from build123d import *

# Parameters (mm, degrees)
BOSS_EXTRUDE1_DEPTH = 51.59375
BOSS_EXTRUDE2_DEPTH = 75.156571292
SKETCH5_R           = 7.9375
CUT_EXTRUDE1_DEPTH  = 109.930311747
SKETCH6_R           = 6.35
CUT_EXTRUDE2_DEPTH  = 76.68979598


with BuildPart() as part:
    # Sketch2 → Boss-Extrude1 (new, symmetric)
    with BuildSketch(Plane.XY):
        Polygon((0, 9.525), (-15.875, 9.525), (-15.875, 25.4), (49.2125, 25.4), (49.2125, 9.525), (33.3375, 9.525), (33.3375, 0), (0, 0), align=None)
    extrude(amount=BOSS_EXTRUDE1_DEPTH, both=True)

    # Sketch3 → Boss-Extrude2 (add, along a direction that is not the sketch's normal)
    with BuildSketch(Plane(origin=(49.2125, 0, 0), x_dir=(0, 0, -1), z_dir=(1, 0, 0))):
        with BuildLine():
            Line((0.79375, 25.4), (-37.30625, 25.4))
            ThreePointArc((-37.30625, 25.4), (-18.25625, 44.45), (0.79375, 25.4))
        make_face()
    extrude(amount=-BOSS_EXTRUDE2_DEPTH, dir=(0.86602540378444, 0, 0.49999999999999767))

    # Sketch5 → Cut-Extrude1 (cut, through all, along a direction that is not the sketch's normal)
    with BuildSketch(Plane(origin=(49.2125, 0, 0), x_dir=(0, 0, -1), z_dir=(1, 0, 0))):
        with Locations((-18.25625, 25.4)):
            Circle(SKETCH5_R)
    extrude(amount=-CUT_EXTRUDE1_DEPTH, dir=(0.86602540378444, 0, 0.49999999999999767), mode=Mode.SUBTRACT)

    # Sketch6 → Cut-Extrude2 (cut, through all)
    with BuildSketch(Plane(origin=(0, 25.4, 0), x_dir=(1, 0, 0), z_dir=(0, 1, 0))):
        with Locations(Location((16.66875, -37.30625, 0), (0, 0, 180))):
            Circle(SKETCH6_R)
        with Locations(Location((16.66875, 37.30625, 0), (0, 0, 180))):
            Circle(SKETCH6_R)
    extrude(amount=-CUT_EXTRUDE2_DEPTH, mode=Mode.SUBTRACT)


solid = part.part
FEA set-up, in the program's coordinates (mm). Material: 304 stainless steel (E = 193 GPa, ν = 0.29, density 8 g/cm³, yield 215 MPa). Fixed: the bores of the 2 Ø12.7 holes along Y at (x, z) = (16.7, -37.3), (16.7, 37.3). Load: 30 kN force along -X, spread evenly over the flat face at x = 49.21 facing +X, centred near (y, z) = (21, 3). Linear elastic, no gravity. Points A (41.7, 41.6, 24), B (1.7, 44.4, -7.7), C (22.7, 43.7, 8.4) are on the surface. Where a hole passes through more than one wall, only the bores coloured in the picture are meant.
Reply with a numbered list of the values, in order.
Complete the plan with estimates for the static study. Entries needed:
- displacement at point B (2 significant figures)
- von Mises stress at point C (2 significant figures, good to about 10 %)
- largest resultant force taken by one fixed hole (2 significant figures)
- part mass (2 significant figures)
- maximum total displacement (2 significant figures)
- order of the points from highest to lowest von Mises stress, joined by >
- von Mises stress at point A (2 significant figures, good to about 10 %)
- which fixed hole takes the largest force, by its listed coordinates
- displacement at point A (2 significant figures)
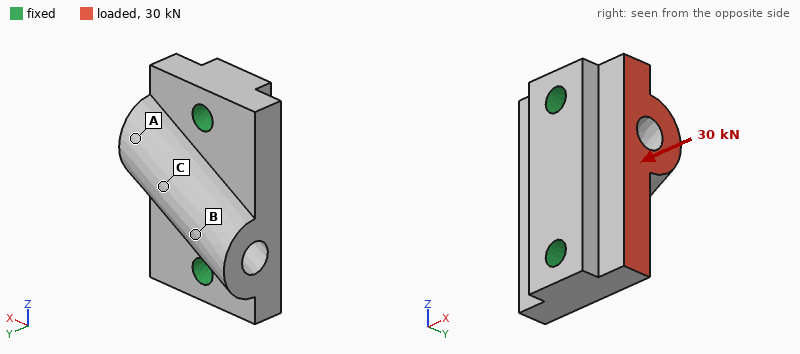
1. 8.6 µm
2. 14 MPa
3. 16 kN
4. 1.3 kg
5. 17 µm
6. A > C > B
7. 28 MPa
8. (16.7, 37.3)
9. 14 µm
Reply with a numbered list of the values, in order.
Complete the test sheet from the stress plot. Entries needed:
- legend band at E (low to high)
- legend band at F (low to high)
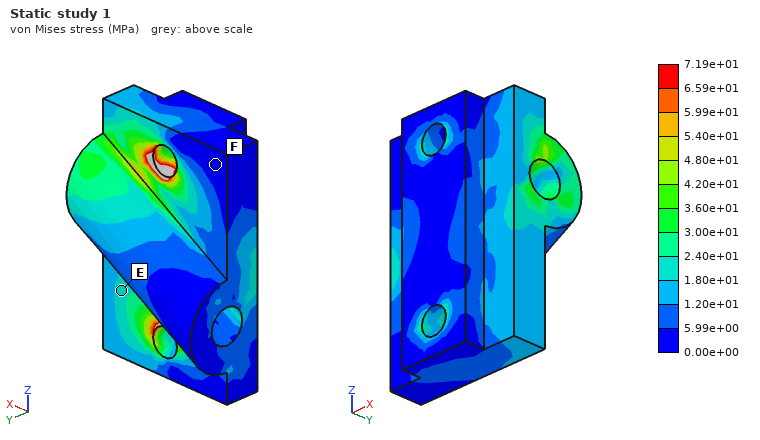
1. 1.80e+01 to 2.40e+01 MPa
2. 0.00e+00 to 5.99e+00 MPa
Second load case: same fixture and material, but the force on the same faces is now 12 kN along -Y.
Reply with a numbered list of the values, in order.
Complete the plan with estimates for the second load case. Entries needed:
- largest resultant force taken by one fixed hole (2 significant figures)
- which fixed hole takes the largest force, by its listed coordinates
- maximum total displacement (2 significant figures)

1. 6.5 kN
2. (16.7, 37.3)
3. 18 µm
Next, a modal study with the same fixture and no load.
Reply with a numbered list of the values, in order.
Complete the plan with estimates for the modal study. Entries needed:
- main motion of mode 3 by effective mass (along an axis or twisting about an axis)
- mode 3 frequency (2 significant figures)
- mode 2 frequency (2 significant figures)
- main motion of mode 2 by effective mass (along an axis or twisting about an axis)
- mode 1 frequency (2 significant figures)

1. along X
2. 14 kHz
3. 12 kHz
4. along Y
5. 8300 Hz
